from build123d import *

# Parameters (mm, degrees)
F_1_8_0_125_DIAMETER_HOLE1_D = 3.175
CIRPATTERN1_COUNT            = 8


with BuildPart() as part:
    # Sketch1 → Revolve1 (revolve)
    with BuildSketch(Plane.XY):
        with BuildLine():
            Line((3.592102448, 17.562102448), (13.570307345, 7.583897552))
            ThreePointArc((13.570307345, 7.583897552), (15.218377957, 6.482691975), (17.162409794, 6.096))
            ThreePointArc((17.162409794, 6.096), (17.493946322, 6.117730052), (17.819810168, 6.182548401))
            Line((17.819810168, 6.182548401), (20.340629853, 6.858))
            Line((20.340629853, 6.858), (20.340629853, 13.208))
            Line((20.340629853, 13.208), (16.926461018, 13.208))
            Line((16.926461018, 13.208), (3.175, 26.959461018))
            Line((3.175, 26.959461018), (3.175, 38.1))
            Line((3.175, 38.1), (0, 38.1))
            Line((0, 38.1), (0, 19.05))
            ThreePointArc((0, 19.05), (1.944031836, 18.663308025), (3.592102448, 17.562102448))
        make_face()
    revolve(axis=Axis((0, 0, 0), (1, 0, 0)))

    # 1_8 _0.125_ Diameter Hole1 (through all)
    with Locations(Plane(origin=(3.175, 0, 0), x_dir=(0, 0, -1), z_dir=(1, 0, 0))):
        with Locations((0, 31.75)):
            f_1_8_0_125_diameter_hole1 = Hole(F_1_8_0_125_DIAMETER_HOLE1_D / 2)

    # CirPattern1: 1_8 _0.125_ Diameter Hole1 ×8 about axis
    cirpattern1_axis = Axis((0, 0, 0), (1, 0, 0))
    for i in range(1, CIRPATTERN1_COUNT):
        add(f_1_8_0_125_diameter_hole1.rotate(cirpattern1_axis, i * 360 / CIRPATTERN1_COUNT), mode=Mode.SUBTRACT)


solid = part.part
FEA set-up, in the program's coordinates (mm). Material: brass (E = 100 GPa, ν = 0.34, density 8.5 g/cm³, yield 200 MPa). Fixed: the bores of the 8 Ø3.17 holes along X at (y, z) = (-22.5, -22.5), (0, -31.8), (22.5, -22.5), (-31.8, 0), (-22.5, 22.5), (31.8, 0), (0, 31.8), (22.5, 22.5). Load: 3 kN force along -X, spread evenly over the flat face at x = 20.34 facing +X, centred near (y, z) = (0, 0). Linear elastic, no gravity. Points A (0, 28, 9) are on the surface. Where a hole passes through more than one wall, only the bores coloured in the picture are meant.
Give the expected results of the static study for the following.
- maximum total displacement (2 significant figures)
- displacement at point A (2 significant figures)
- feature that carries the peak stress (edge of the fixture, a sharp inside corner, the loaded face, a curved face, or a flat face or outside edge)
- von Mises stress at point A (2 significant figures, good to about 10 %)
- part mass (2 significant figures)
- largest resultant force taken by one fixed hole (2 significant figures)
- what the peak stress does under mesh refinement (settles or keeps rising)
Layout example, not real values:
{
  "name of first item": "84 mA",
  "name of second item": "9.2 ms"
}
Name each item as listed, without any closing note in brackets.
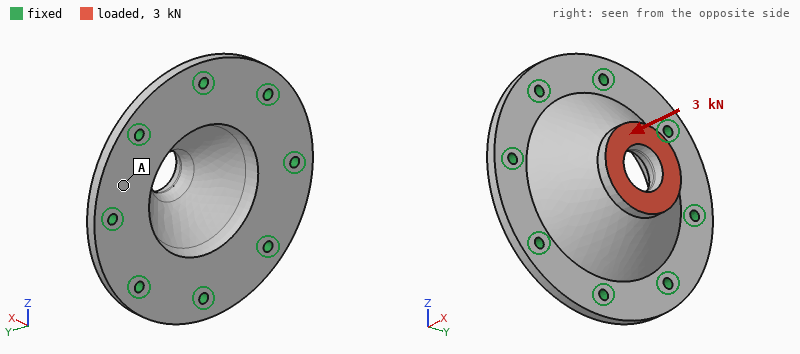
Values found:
{
  "maximum total displacement": "8.2 µm",
  "displacement at point A": "3.5 µm",
  "feature that carries the peak stress": "edge of the fixture",
  "von Mises stress at point A": "8.9 MPa",
  "part mass": "210 g",
  "largest resultant force taken by one fixed hole": "590 N",
  "what the peak stress does under mesh refinement": "keeps rising"
}
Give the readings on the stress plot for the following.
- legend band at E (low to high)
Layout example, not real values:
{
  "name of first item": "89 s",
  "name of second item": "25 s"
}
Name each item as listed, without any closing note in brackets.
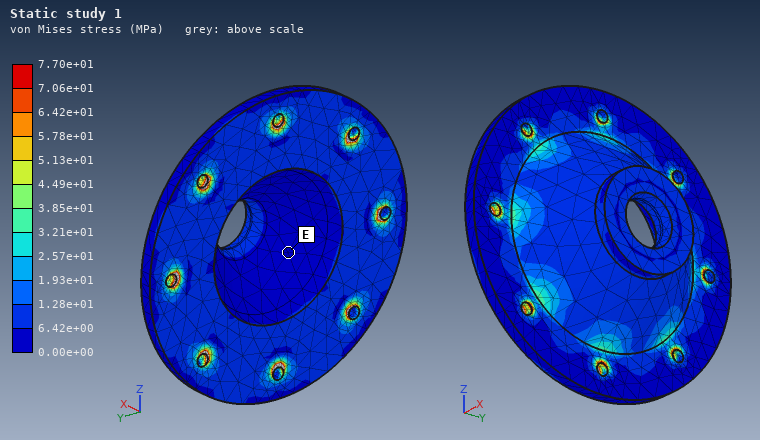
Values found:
{
  "legend band at E": "0.00e+00 to 6.42e+00 MPa"
}
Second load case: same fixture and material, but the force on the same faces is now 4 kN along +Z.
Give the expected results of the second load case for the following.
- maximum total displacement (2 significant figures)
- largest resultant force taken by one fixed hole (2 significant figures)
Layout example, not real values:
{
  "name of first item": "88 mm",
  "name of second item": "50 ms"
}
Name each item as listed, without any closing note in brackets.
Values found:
{
  "maximum total displacement": "13 µm",
  "largest resultant force taken by one fixed hole": "1.1 kN"
}
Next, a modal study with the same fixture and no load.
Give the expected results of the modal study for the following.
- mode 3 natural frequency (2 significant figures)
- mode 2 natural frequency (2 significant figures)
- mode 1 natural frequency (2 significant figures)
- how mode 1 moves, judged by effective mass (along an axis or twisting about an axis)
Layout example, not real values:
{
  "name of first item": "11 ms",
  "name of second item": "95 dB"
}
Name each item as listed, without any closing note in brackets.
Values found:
{
  "mode 3 natural frequency": "12 kHz",
  "mode 2 natural frequency": "12 kHz",
  "mode 1 natural frequency": "9000 Hz",
  "how mode 1 moves, judged by effective mass": "along X"
}
